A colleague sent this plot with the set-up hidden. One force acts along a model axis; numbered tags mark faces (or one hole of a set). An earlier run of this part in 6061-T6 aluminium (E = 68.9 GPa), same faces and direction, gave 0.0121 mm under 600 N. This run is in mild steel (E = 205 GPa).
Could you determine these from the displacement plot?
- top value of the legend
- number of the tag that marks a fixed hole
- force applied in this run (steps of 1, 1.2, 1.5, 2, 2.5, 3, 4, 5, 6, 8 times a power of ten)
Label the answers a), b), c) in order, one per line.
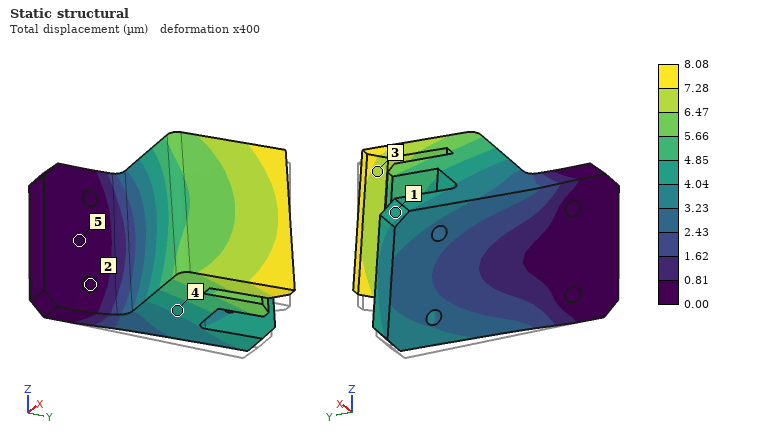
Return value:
a) 8.08 µm
b) 2
c) 1.2 kN
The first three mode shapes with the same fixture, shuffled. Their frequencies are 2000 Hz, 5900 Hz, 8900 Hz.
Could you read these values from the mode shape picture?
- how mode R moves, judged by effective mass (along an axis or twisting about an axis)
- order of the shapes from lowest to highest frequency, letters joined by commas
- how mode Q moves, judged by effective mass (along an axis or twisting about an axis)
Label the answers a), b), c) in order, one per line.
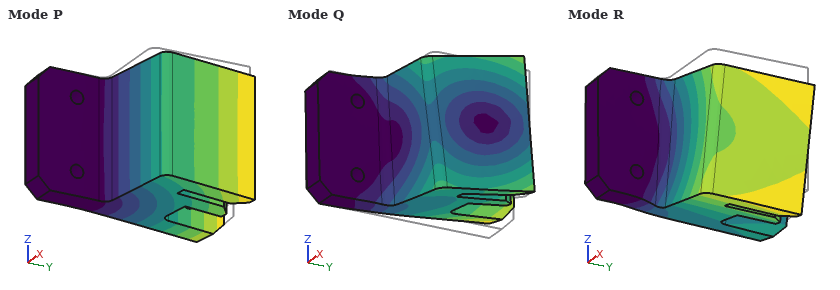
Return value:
a) along Z
b) P, R, Q
c) along Z
